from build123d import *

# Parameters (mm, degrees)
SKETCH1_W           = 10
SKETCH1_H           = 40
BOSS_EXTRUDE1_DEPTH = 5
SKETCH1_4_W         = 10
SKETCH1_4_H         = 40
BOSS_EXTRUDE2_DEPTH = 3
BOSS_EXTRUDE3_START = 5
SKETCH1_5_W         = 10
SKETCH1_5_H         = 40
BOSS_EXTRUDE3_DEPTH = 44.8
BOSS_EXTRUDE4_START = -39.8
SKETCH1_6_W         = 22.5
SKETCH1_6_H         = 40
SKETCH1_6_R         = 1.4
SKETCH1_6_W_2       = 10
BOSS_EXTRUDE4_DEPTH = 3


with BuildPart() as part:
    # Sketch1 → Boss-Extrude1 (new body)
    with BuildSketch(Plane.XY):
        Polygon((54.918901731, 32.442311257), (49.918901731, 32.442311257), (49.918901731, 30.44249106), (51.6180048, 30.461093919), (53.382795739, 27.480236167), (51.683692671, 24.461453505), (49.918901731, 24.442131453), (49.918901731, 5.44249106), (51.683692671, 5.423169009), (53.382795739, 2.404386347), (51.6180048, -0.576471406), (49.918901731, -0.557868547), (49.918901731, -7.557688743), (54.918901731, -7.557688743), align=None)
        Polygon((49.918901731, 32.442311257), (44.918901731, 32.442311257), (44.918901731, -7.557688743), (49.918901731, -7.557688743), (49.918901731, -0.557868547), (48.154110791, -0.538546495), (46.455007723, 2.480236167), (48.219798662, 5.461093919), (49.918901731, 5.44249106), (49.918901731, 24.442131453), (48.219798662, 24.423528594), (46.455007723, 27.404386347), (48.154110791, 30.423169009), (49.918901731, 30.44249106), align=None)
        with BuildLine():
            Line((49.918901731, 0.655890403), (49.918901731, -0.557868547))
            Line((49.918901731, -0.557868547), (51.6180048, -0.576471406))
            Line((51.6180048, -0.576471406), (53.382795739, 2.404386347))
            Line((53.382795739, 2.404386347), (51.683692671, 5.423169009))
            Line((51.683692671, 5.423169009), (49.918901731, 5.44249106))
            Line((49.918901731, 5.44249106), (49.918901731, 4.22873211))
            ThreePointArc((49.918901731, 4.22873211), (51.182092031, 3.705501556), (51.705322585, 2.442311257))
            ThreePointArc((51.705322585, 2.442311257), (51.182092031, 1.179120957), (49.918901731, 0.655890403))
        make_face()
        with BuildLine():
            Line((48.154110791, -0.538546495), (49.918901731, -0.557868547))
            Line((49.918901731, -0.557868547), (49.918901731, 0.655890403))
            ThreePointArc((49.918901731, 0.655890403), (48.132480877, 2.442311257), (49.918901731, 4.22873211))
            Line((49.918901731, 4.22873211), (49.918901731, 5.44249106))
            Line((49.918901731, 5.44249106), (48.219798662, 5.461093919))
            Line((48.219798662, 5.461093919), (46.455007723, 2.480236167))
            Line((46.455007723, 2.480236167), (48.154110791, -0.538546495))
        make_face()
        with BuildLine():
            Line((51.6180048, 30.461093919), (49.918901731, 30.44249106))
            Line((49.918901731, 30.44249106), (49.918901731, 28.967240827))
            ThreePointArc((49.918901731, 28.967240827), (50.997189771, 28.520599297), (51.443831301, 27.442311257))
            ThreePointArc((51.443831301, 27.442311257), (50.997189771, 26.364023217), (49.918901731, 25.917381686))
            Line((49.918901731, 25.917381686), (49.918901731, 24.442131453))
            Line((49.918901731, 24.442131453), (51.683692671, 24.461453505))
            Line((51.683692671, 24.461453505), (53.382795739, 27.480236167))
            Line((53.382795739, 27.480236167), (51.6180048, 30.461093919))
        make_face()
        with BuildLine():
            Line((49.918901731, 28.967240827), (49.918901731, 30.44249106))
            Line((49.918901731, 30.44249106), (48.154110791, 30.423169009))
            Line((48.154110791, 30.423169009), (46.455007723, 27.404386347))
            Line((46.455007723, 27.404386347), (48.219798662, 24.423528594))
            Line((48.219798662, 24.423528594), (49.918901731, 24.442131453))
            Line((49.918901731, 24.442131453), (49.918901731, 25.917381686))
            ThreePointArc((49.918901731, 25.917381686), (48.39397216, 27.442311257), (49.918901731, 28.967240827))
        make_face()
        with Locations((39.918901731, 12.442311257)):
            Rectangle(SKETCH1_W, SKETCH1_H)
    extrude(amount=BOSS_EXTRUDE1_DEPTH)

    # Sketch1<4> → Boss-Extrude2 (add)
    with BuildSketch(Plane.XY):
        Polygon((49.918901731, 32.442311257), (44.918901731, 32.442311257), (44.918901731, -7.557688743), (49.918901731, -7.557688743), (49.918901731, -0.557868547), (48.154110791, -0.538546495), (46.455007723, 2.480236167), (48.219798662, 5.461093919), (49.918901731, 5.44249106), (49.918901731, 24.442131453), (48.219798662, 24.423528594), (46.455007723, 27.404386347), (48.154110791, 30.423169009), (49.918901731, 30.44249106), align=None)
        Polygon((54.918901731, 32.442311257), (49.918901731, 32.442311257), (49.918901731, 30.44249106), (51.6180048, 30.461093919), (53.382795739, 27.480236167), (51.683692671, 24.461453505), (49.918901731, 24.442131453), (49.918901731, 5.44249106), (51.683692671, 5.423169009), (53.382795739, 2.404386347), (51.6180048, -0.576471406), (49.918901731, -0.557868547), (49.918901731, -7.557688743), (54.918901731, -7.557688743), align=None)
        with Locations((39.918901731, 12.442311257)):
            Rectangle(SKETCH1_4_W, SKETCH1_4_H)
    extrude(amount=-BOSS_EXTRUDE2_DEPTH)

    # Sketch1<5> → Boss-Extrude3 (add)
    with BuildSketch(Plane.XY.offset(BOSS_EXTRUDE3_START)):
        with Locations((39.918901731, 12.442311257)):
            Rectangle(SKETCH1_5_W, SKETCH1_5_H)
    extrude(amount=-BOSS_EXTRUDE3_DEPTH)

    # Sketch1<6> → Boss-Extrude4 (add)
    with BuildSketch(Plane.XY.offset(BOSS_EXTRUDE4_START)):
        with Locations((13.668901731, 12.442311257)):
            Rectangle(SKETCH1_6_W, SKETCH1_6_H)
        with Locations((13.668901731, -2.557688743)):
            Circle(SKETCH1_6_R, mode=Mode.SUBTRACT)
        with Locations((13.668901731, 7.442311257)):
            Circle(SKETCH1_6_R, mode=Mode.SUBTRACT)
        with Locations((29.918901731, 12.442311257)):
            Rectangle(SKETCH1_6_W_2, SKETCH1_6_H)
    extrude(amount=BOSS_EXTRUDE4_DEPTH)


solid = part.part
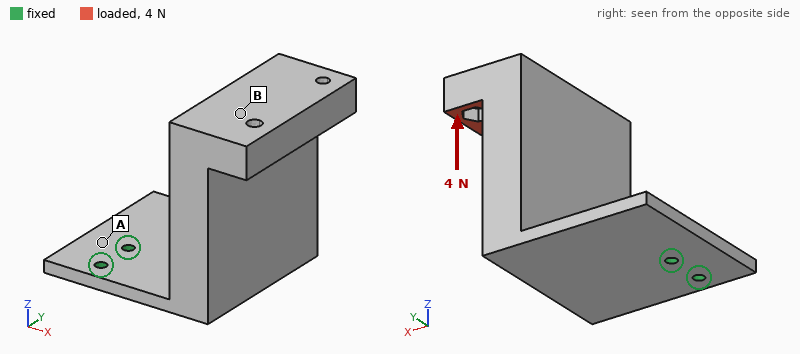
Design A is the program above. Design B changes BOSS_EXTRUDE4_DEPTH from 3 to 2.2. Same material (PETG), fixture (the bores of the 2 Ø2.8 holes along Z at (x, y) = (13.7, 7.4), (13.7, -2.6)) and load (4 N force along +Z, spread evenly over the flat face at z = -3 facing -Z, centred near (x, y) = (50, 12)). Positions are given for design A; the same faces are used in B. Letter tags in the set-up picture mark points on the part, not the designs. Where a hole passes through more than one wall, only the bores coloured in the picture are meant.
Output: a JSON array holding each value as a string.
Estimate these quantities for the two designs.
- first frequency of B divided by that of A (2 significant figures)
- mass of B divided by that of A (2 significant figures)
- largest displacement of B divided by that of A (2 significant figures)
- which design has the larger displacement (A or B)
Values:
["0.64", "0.96", "2.4", "B"]
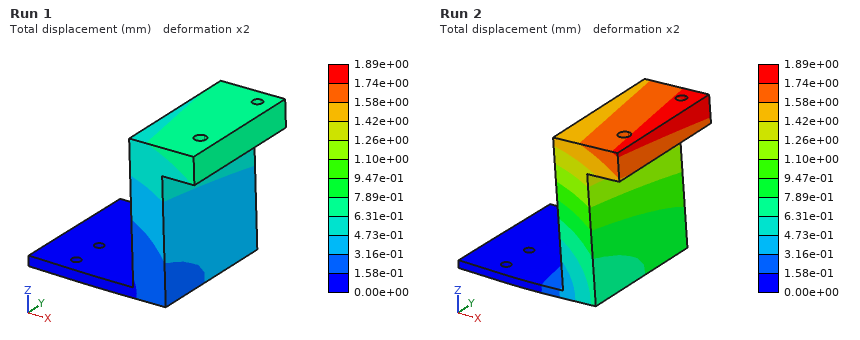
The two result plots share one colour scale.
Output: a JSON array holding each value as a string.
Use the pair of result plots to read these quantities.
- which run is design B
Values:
["Run 2"]
